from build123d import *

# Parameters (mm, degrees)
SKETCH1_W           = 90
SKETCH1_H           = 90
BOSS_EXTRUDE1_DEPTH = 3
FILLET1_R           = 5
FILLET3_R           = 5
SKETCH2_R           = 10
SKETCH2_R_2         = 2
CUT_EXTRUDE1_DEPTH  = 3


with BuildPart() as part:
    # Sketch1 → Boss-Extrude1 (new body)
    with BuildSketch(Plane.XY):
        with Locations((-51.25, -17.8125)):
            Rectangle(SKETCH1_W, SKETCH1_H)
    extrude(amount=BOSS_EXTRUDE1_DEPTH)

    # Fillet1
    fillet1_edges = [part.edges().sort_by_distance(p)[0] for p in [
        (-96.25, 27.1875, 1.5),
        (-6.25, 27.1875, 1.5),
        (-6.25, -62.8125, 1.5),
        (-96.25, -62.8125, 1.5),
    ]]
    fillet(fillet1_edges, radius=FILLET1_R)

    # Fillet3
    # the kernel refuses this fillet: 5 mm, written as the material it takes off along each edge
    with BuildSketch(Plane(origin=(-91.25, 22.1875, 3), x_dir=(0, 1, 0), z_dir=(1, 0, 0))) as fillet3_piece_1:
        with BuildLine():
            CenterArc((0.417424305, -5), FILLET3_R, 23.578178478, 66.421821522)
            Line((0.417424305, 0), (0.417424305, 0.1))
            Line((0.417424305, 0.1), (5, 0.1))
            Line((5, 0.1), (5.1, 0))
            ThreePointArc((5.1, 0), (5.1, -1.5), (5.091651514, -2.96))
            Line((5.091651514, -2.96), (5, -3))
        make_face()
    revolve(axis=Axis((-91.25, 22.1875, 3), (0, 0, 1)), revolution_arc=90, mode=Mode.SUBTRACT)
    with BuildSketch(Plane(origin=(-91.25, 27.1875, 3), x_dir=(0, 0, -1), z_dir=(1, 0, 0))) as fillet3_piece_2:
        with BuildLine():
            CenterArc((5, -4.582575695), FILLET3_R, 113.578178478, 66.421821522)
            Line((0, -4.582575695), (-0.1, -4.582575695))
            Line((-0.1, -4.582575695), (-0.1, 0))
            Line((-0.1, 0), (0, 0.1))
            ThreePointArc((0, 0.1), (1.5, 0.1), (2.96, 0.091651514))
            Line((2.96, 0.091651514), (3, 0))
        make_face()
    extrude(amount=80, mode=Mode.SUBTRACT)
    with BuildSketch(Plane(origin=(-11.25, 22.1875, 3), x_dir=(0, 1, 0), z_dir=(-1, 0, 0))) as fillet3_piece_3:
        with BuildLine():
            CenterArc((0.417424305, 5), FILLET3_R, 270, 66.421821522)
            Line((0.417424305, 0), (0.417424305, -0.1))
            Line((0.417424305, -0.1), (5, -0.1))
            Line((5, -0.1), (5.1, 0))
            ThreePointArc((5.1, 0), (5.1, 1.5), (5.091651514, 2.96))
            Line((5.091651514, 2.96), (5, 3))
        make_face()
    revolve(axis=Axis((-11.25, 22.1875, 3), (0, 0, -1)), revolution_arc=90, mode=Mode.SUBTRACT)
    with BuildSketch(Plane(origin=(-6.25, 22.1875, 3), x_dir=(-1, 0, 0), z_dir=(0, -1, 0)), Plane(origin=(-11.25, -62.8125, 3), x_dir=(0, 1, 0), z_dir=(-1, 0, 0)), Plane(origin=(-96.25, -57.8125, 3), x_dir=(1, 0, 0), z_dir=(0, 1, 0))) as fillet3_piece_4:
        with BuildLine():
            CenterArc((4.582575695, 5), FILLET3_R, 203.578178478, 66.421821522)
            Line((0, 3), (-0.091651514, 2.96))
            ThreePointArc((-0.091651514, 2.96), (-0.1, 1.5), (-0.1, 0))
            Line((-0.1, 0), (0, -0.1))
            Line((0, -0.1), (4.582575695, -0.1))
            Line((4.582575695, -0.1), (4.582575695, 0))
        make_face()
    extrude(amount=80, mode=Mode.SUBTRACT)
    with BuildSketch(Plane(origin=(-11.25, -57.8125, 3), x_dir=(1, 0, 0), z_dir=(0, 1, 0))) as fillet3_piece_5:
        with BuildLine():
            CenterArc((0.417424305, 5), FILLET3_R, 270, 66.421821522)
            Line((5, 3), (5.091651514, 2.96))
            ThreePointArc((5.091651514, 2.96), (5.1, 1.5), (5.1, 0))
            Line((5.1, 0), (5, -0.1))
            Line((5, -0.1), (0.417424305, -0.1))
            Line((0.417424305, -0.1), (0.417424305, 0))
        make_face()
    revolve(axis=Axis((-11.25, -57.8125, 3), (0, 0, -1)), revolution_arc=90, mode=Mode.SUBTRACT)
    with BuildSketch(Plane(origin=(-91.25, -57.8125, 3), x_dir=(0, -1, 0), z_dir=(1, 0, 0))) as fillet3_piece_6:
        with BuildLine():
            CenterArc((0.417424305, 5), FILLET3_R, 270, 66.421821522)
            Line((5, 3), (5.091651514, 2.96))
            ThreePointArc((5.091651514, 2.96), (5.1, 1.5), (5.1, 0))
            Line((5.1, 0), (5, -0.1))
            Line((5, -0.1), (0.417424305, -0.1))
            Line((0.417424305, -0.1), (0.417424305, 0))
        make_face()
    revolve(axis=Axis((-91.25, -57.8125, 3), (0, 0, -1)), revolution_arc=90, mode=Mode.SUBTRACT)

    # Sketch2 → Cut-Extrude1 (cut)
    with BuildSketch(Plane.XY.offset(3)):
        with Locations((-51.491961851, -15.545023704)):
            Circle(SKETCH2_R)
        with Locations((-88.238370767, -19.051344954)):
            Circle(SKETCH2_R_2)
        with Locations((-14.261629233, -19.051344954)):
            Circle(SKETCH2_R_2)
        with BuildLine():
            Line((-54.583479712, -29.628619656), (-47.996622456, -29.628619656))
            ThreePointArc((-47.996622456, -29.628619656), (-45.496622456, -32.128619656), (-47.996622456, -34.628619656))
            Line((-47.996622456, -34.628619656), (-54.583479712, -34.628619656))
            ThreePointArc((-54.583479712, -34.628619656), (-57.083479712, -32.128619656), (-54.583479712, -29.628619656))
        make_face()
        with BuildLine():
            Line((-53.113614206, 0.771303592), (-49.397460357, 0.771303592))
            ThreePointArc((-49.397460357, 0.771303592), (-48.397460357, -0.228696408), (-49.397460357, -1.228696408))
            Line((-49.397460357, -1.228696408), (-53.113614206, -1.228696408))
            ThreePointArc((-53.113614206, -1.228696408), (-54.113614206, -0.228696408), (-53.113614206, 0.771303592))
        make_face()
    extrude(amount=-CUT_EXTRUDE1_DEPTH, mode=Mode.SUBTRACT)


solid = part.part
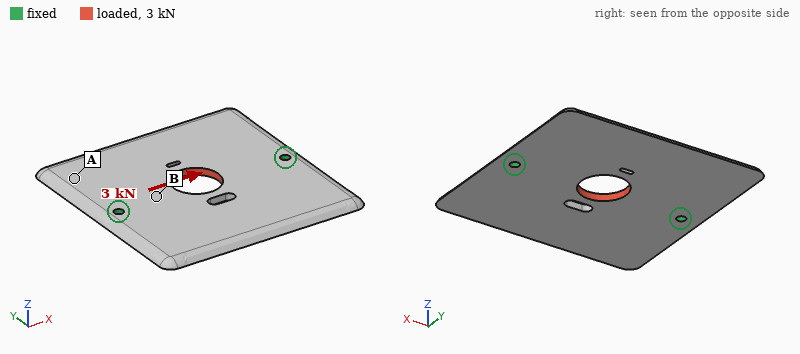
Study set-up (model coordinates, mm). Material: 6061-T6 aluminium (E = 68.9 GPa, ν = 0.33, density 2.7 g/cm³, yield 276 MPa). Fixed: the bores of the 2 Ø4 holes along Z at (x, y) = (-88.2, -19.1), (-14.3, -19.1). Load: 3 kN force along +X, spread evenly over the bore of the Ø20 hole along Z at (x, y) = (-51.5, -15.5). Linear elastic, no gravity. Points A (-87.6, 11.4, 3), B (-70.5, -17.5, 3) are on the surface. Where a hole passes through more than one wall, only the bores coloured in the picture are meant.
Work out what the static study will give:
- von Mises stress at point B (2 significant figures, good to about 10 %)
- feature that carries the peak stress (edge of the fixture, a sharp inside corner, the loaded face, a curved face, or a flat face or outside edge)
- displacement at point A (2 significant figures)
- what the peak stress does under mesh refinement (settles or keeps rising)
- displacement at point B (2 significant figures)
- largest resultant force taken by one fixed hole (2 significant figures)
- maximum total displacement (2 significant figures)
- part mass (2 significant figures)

21 MPa
edge of the fixture
9.2 µm
keeps rising
7.2 µm
1.5 kN
13 µm
59 g
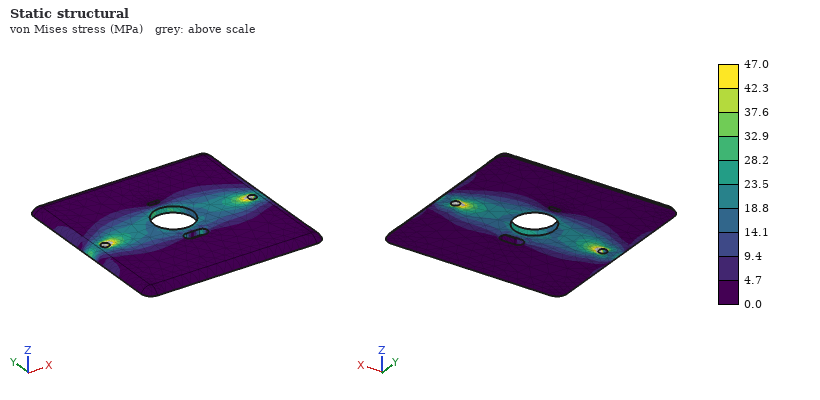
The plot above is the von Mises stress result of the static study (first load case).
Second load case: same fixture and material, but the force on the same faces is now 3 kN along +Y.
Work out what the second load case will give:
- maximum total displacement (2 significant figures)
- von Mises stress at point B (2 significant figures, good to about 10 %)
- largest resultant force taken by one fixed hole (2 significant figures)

20 µm
13 MPa
1.5 kN
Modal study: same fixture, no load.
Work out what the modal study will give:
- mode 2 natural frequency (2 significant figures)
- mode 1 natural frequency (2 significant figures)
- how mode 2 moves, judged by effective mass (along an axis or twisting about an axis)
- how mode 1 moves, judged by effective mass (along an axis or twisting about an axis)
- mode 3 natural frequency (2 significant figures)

1100 Hz
820 Hz
along Z
twisting about X
1800 Hz
